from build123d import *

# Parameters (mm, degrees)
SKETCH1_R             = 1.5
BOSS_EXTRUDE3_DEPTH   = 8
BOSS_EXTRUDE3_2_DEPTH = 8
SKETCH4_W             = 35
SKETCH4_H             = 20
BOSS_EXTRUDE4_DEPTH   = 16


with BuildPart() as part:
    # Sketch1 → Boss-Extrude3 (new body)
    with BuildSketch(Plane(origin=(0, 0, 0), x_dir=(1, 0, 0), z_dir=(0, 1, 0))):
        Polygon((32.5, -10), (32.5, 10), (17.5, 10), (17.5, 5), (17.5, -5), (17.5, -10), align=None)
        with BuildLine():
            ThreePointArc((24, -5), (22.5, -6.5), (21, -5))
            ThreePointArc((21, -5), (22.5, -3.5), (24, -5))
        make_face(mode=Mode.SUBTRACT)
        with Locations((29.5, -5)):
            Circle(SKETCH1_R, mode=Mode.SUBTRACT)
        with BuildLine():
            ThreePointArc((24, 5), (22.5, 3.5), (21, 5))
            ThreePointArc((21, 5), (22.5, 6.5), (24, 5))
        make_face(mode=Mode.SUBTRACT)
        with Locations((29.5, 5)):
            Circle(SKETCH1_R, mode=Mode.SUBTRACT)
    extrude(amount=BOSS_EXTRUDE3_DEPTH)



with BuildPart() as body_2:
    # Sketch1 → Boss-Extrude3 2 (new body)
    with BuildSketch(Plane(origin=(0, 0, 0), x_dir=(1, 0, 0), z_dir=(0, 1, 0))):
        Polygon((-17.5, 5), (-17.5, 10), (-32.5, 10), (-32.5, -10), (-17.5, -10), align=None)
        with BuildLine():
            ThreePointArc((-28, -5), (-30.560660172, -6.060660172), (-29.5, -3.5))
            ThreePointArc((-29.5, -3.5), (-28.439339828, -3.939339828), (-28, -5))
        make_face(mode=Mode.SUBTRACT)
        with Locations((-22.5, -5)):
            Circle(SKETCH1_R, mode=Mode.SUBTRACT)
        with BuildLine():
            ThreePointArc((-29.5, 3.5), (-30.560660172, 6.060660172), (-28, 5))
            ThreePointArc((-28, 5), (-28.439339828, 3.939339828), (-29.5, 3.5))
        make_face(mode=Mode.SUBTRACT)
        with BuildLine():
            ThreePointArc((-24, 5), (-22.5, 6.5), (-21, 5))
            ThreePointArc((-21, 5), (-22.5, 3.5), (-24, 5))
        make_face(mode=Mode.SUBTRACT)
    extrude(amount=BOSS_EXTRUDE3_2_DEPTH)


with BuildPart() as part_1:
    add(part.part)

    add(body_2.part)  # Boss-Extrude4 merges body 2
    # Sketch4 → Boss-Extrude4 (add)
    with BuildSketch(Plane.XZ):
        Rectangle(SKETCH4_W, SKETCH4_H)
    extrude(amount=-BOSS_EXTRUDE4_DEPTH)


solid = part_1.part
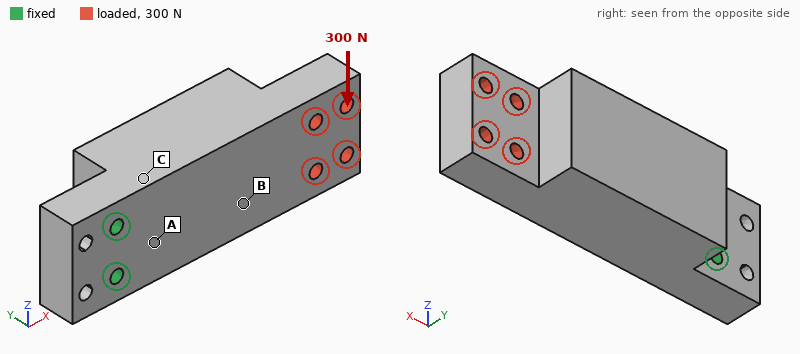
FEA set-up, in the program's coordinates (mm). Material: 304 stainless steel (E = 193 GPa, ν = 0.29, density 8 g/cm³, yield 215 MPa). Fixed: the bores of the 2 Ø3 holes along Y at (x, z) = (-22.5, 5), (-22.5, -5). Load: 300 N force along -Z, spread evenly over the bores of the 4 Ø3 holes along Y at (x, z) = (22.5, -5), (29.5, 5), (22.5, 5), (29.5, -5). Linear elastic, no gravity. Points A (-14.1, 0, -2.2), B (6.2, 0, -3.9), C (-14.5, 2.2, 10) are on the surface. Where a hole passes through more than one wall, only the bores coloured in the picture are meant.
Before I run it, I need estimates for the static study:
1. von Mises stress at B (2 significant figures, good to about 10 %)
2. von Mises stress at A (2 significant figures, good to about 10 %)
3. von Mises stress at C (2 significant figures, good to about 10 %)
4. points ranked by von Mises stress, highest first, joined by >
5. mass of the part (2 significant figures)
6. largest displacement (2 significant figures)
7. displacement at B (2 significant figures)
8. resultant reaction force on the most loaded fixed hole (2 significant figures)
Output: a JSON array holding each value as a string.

["4.6 MPa", "11 MPa", "18 MPa", "C > A > B", "120 g", "14 µm", "5.7 µm", "1.2 kN"]
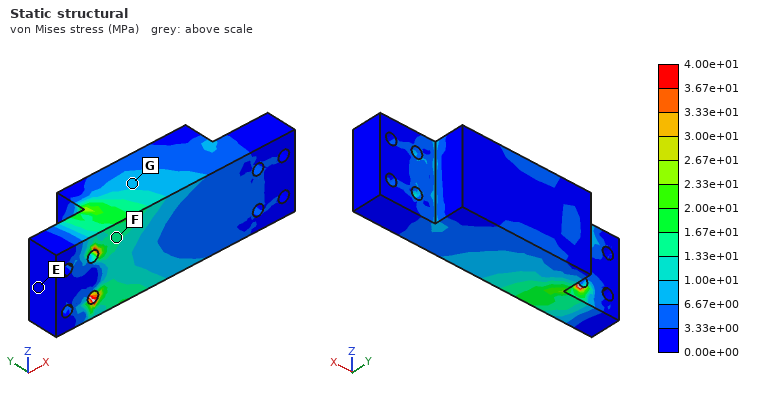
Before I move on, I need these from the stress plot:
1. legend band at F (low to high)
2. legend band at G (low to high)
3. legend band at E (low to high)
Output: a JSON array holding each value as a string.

["1.33e+01 to 1.67e+01 MPa", "6.67e+00 to 1.00e+01 MPa", "0.00e+00 to 3.33e+00 MPa"]
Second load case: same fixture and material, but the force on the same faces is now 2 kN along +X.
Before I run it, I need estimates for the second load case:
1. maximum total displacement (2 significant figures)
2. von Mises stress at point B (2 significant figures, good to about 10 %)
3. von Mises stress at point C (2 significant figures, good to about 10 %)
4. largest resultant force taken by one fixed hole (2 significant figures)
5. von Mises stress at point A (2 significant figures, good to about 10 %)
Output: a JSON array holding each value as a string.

["7.6 µm", "16 MPa", "12 MPa", "1.0 kN", "15 MPa"]
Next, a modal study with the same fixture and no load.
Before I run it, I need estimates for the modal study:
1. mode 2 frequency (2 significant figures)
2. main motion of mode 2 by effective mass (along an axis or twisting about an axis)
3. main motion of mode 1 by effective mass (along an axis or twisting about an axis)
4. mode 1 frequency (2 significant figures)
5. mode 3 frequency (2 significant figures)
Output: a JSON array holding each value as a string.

["4500 Hz", "along Z", "along Y", "2400 Hz", "11 kHz"]
